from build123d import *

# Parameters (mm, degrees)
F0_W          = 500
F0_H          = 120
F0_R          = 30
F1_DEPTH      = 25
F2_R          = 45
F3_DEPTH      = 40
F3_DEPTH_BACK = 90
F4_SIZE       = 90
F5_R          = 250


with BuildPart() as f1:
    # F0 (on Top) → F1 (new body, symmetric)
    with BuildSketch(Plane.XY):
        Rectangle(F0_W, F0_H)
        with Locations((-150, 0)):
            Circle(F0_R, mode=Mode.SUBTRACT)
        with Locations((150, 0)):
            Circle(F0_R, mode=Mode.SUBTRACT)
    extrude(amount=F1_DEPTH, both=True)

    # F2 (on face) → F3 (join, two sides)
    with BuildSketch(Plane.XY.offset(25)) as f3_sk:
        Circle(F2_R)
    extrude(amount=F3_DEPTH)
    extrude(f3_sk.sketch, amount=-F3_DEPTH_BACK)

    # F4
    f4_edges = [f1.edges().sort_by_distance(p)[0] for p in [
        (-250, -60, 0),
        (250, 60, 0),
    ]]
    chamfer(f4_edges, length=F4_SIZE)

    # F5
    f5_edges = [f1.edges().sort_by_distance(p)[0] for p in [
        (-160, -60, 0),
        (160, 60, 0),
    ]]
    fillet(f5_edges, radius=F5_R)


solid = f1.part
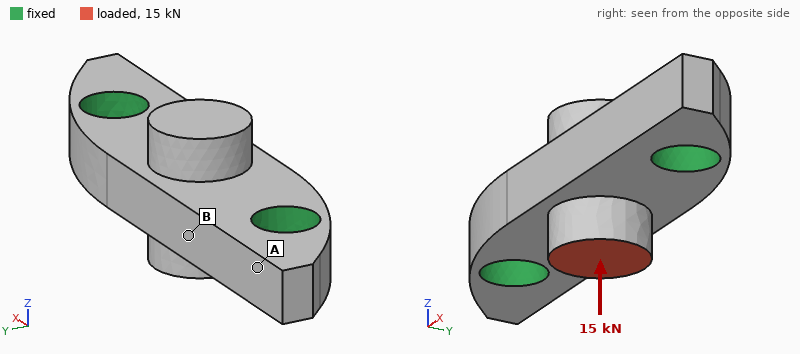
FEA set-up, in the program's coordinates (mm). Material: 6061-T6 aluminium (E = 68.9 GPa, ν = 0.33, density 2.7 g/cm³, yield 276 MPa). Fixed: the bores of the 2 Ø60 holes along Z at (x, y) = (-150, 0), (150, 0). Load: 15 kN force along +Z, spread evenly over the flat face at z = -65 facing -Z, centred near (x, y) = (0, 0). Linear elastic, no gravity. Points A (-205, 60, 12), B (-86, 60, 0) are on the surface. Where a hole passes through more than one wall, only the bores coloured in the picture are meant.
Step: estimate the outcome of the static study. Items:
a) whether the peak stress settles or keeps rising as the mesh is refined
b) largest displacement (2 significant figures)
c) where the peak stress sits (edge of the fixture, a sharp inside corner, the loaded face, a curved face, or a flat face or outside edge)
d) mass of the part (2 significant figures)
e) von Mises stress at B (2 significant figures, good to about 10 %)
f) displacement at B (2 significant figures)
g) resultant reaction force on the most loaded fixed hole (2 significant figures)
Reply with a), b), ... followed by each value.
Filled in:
a) keeps rising
b) 16 µm
c) edge of the fixture
d) 7.3 kg
e) 2.8 MPa
f) 5.8 µm
g) 7.5 kN
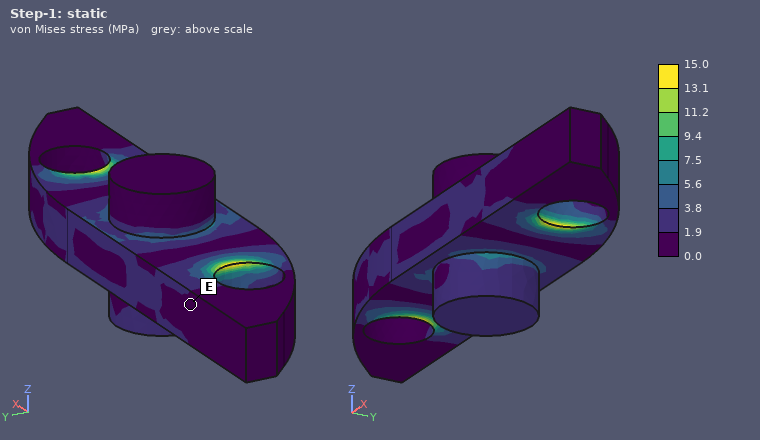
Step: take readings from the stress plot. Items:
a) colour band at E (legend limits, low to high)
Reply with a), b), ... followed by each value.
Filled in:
a) 0.0 to 1.9 MPa
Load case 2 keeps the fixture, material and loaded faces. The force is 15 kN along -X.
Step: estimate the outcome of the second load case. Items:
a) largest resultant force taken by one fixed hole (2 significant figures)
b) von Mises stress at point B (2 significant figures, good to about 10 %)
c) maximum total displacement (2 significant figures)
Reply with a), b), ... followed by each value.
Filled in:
a) 9.0 kN
b) 2.0 MPa
c) 19 µm
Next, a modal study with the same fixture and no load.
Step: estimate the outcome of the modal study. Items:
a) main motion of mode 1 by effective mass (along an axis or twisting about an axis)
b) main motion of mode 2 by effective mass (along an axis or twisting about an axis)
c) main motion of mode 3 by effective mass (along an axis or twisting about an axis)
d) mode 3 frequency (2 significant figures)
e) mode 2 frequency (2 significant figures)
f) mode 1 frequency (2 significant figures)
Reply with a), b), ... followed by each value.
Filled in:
a) along Z
b) twisting about X
c) along Y
d) 3300 Hz
e) 2900 Hz
f) 2700 Hz
